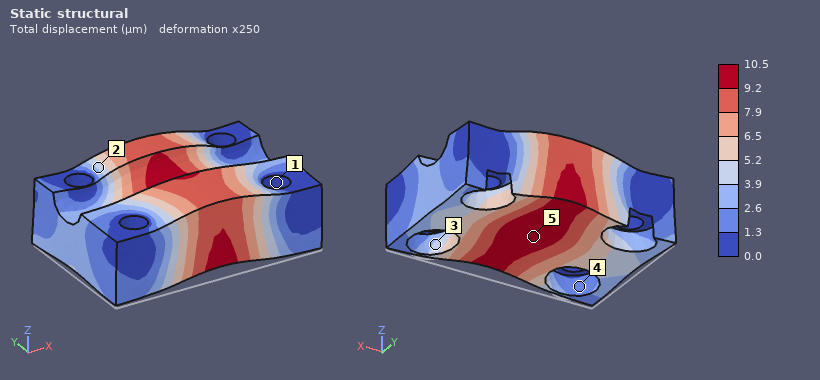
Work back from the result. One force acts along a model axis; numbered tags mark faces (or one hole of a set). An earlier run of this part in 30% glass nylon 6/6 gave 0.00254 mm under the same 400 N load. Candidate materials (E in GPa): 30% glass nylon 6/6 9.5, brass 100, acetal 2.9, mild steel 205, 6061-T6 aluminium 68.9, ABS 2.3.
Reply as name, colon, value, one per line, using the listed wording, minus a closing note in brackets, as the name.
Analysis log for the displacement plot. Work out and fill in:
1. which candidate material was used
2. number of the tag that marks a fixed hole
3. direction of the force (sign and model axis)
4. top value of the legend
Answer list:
which candidate material was used: ABS
number of the tag that marks a fixed hole: 1
direction of the force: +Z
top value of the legend: 10.5 µm
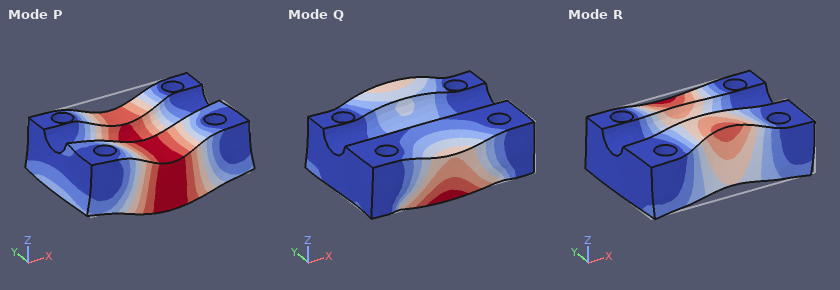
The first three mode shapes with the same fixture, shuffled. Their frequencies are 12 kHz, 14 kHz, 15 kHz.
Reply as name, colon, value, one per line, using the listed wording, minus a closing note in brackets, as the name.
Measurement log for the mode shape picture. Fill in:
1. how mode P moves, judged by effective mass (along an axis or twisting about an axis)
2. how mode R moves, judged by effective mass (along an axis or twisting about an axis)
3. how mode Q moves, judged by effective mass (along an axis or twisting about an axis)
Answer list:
how mode P moves, judged by effective mass: along Z
how mode R moves, judged by effective mass: along Y
how mode Q moves, judged by effective mass: along Y
